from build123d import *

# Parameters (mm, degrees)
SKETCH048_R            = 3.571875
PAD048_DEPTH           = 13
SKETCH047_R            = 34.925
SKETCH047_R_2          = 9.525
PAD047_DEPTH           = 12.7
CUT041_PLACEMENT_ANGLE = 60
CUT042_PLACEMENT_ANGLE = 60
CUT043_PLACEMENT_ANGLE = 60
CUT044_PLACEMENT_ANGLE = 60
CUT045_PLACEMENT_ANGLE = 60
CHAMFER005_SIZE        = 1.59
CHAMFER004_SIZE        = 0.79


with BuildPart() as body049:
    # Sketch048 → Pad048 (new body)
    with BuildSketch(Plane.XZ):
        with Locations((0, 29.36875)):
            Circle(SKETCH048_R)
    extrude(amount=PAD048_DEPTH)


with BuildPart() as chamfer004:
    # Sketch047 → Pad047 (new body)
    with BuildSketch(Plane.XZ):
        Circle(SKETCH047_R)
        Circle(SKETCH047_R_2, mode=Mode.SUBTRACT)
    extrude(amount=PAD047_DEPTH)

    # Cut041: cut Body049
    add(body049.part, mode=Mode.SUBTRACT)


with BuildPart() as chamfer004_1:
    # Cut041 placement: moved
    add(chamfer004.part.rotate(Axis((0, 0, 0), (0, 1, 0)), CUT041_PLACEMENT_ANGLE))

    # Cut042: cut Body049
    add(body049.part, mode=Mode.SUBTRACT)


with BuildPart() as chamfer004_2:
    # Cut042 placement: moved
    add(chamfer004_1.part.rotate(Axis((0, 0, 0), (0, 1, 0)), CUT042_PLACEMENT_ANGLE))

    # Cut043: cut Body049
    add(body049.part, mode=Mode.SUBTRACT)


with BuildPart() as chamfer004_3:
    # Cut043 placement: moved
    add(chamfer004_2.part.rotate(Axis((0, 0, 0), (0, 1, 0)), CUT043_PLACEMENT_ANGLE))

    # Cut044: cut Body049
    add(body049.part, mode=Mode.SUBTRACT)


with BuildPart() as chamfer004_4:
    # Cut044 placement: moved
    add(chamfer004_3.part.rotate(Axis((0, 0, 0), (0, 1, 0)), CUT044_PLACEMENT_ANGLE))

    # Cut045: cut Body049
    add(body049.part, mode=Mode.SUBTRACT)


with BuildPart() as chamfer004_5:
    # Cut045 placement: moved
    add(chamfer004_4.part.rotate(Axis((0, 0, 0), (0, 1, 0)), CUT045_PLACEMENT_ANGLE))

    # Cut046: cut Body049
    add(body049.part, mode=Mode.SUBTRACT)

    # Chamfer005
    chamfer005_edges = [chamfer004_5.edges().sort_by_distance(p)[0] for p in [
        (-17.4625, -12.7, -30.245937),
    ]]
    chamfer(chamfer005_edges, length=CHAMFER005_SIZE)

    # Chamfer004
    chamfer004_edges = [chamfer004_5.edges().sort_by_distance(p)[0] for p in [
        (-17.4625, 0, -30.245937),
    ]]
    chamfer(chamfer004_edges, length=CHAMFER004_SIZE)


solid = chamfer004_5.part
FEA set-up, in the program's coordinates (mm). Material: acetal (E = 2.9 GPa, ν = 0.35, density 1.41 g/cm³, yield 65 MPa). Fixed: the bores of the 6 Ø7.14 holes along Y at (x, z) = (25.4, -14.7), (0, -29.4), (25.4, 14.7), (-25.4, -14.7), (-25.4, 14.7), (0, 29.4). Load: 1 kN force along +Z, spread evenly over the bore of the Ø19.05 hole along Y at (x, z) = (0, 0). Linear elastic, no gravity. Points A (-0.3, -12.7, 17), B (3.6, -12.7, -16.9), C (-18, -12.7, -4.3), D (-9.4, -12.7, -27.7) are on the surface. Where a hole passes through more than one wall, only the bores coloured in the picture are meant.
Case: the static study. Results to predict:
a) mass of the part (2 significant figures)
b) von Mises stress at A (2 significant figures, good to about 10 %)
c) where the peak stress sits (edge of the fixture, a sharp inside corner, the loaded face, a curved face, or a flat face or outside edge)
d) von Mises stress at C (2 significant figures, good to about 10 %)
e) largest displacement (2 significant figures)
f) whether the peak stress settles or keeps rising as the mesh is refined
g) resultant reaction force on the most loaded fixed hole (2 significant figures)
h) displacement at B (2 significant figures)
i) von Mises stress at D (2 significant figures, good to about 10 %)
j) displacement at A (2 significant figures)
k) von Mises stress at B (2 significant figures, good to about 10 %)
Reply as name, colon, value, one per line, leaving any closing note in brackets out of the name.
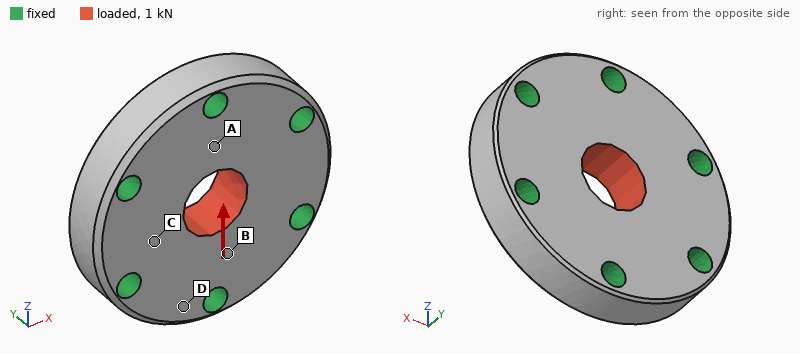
mass of the part: 59 g
von Mises stress at A: 1.5 MPa
where the peak stress sits: edge of the fixture
von Mises stress at C: 0.68 MPa
largest displacement: 8.8 µm
whether the peak stress settles or keeps rising as the mesh is refined: keeps rising
resultant reaction force on the most loaded fixed hole: 260 N
displacement at B: 5.1 µm
von Mises stress at D: 0.43 MPa
displacement at A: 5.1 µm
von Mises stress at B: 1.3 MPa
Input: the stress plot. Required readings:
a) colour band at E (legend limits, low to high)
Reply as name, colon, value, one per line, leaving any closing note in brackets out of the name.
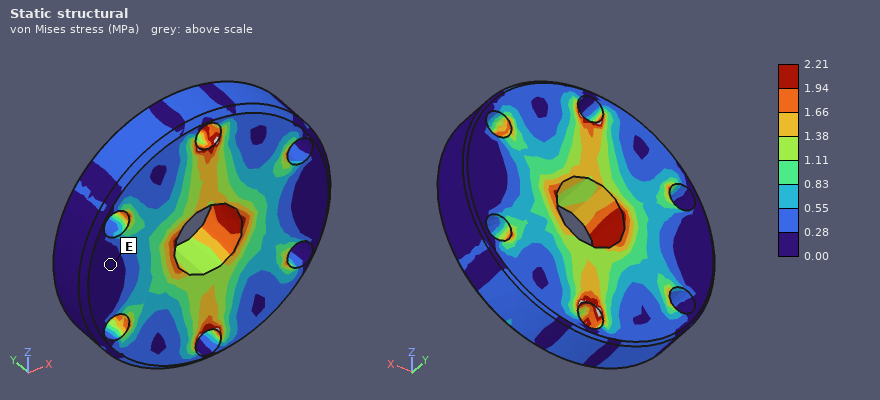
colour band at E: 0.00 to 0.28 MPa
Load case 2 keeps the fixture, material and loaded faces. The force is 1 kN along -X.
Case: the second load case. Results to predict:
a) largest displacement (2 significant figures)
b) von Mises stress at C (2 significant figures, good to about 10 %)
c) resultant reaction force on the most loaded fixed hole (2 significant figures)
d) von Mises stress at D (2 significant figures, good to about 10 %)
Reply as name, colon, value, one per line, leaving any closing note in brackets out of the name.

largest displacement: 8.9 µm
von Mises stress at C: 0.92 MPa
resultant reaction force on the most loaded fixed hole: 230 N
von Mises stress at D: 0.26 MPa
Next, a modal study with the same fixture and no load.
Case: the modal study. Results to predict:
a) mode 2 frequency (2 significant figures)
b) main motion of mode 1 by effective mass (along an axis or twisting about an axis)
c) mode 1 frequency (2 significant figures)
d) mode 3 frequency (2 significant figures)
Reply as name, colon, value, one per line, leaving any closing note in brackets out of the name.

mode 2 frequency: 11 kHz
main motion of mode 1 by effective mass: along Y
mode 1 frequency: 7900 Hz
mode 3 frequency: 11 kHz
